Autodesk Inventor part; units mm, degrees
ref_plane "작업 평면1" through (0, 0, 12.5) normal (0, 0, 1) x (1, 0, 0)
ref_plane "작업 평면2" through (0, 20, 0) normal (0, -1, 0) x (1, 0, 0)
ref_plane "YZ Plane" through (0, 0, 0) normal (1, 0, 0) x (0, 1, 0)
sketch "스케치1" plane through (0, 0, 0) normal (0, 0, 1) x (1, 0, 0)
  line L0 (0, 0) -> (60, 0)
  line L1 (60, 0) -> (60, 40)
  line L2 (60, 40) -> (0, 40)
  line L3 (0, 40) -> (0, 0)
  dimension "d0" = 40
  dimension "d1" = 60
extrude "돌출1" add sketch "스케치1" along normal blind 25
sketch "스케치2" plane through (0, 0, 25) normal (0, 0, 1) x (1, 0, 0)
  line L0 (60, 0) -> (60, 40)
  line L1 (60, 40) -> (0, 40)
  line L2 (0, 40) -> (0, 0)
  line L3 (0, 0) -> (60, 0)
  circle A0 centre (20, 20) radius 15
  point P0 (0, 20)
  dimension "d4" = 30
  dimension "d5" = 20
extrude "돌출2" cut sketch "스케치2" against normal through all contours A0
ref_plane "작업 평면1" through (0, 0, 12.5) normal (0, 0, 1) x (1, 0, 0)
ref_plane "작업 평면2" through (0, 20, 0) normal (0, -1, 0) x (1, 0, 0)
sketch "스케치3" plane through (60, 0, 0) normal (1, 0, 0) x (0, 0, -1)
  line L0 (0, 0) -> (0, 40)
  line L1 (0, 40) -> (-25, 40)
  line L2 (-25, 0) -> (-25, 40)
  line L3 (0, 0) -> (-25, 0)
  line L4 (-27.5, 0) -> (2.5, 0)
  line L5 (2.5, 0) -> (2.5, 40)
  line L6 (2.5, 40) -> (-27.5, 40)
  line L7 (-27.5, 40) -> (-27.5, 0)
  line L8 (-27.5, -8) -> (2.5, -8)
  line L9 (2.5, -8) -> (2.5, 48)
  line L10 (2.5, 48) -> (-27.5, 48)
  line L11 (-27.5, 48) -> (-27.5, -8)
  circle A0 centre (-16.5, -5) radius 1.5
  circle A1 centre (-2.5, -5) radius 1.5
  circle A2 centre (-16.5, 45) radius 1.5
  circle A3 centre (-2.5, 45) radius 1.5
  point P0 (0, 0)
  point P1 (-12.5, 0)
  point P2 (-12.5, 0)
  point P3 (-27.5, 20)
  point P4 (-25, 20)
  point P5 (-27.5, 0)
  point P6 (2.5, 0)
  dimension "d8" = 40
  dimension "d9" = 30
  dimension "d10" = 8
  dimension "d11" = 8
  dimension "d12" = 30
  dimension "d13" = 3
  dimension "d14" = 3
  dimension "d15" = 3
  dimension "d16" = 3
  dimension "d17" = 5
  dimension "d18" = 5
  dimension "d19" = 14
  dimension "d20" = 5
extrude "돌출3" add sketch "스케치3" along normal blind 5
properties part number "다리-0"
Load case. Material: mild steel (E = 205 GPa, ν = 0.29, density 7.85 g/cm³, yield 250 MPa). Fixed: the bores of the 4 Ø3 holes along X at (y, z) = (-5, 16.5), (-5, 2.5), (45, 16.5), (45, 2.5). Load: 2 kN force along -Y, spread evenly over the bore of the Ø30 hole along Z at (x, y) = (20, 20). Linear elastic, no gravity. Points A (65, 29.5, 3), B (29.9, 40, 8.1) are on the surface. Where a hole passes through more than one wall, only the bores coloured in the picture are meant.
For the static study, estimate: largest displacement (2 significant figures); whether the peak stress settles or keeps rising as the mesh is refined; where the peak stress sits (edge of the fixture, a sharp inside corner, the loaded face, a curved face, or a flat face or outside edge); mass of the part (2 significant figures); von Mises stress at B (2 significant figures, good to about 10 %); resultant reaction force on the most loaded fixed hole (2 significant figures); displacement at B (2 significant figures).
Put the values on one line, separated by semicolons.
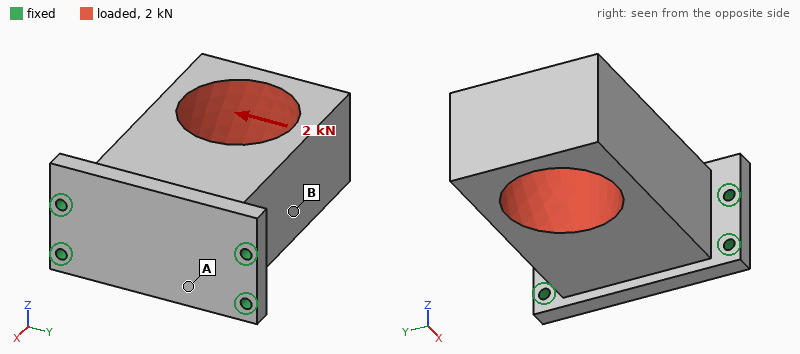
22 µm; keeps rising; edge of the fixture; 400 g; 21 MPa; 1.2 kN; 8.7 µm
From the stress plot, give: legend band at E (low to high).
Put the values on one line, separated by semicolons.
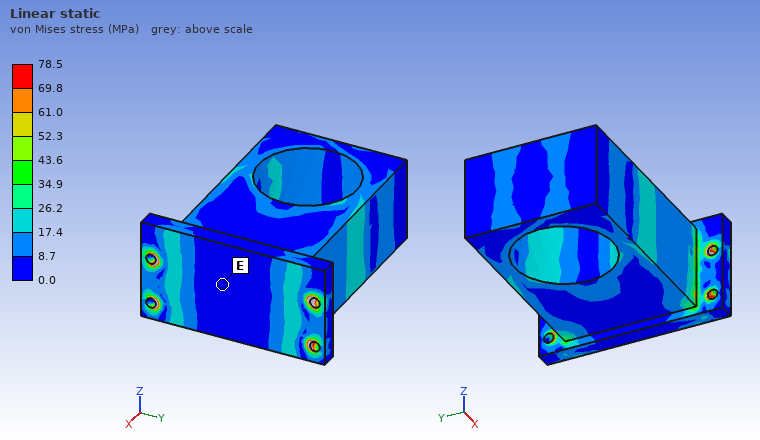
0.0 to 8.7 MPa
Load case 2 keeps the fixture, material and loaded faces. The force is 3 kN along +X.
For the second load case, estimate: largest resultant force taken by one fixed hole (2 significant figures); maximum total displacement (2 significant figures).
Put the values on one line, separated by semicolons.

1.1 kN; 8.8 µm
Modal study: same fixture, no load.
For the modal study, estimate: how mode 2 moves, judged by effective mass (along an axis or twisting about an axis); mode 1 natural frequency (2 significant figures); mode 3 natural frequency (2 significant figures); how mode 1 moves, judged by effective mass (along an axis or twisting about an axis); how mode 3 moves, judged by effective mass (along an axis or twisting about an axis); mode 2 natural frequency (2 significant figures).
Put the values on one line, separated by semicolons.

along Y; 2000 Hz; 8000 Hz; along Z; along X; 4100 Hz
